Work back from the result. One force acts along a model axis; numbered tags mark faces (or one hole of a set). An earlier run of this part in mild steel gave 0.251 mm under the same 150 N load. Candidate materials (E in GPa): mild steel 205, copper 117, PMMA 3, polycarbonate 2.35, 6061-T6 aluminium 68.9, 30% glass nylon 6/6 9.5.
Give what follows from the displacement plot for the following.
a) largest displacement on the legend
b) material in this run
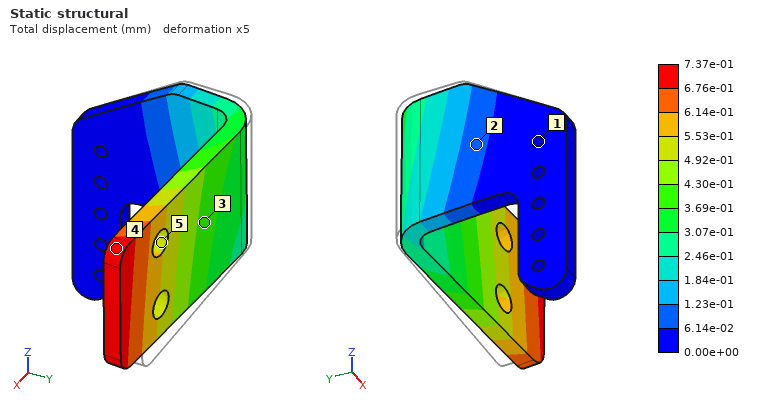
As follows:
7.37e-01 mm
6061-T6 aluminium
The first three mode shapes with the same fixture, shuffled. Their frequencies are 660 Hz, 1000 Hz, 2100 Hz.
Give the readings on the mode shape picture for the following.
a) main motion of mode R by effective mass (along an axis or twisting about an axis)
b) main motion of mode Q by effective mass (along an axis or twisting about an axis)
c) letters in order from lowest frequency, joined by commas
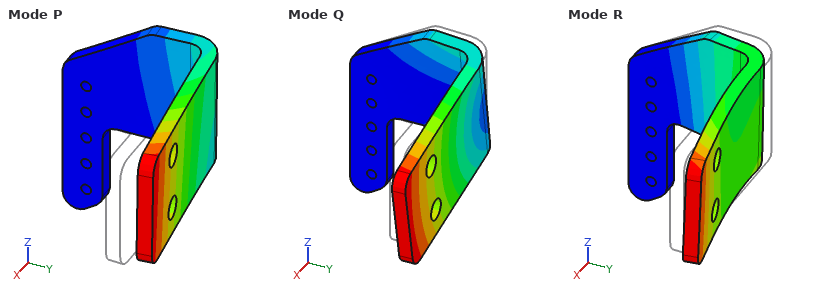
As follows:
along X
along Z
P, Q, R
